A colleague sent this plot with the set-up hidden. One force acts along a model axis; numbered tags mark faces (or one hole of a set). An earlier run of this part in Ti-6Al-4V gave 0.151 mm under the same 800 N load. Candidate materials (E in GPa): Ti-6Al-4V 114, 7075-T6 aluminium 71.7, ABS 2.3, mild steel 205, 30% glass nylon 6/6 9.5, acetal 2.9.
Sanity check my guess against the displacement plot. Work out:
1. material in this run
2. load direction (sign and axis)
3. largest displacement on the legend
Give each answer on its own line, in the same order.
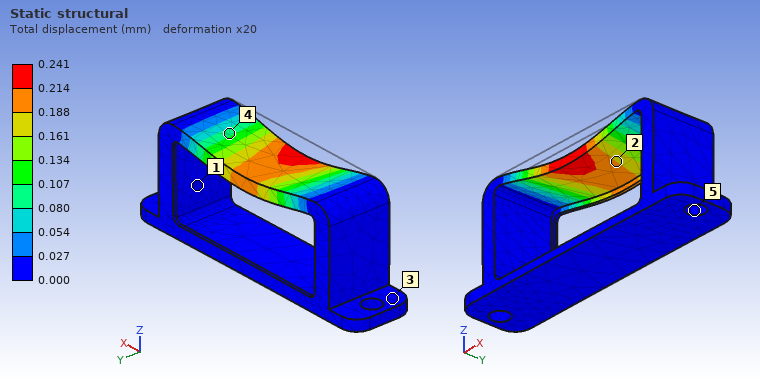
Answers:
7075-T6 aluminium
-Z
0.241 mm
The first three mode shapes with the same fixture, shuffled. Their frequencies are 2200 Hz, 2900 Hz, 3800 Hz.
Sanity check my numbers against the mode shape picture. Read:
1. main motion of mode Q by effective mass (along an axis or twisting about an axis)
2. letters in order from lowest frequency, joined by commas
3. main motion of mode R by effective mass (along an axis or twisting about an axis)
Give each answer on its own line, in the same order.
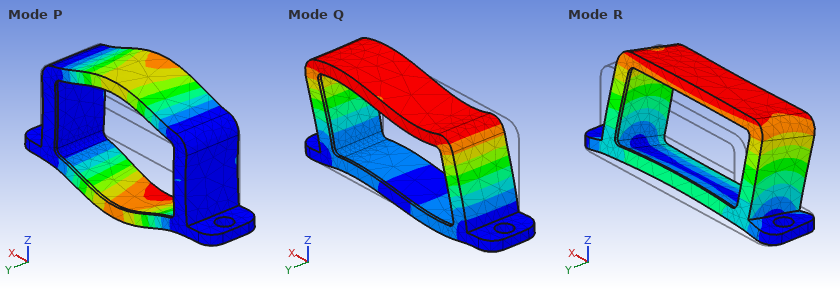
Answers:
along X
Q, R, P
along Y
